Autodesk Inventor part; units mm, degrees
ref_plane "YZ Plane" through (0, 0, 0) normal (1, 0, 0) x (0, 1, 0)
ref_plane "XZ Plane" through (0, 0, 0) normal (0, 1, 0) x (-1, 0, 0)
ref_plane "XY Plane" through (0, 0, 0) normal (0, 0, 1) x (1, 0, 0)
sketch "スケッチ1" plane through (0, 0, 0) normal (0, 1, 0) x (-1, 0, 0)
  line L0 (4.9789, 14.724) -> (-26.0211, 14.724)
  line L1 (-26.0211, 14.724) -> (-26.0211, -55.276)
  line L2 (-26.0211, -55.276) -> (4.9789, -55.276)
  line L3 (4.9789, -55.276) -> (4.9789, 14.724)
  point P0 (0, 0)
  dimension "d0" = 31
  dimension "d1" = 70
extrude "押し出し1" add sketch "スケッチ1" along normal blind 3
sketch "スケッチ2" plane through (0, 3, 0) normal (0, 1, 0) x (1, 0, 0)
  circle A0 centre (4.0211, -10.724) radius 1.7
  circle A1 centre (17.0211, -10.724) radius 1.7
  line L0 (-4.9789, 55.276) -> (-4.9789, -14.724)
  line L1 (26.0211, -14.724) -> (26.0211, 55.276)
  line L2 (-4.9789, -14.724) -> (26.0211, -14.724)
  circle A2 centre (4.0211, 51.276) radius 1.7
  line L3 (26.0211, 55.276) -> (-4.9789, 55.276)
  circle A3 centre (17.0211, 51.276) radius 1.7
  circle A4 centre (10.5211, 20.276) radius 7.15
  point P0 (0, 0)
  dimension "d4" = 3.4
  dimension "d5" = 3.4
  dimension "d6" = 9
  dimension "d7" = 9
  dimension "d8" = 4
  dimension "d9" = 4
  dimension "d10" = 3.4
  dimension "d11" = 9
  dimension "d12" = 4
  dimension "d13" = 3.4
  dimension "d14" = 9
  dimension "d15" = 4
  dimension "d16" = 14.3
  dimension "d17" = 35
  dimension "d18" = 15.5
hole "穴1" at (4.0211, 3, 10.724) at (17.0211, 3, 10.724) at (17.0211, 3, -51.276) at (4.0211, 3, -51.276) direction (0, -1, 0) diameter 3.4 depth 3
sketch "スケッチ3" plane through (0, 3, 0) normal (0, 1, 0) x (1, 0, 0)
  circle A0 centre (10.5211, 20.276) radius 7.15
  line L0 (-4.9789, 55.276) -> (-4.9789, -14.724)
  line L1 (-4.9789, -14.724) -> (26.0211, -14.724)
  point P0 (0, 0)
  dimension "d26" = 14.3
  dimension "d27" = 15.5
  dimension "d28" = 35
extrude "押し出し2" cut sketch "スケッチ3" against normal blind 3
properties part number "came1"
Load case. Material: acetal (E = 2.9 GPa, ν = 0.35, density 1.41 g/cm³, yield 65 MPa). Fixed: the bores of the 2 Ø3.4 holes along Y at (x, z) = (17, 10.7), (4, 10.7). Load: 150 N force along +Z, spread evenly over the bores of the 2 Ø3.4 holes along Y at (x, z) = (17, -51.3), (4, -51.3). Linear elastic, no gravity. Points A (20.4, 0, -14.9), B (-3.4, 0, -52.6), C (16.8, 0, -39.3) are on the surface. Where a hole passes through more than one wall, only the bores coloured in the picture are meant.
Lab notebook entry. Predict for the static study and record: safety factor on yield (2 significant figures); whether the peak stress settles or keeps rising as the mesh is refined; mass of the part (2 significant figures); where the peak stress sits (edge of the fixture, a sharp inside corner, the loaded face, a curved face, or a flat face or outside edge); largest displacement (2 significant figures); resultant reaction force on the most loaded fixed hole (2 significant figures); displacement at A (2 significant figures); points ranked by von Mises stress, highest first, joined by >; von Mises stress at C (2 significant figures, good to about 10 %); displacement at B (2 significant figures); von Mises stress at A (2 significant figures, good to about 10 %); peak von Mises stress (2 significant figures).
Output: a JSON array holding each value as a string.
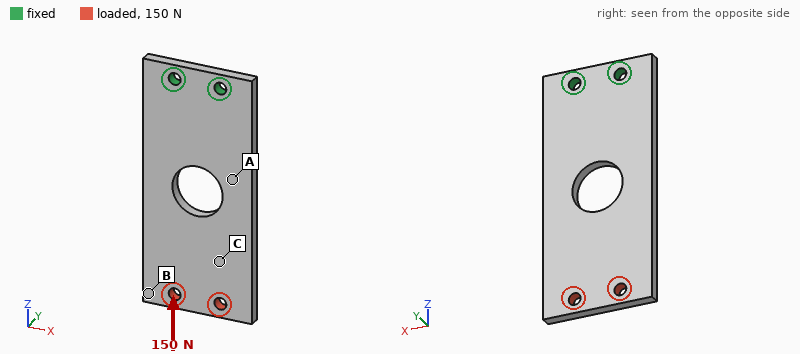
["9.7", "settles", "8.3 g", "a curved face", "56 µm", "75 N", "21 µm", "A > C > B", "1.8 MPa", "44 µm", "2.9 MPa", "6.7 MPa"]
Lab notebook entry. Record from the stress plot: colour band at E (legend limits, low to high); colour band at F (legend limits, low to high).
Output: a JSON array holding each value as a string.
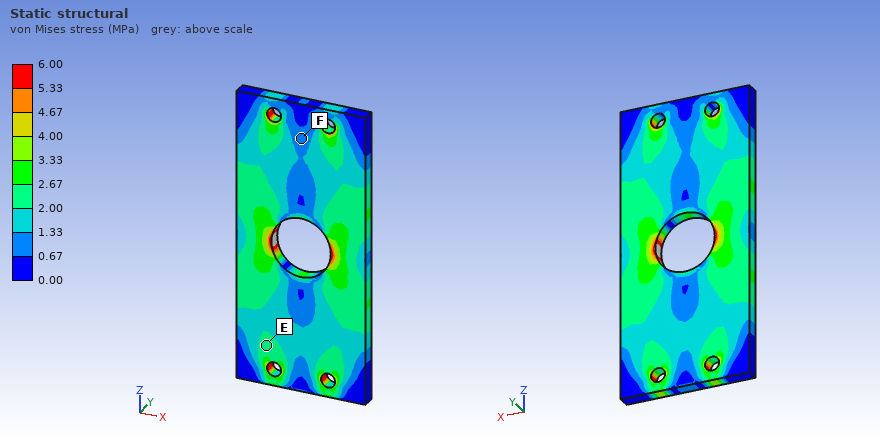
["2.00 to 2.67 MPa", "0.67 to 1.33 MPa"]
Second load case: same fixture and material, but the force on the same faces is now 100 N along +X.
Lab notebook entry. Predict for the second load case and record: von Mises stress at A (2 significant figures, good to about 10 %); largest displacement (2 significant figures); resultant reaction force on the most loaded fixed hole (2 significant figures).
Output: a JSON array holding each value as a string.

["6.4 MPa", "0.80 mm", "390 N"]
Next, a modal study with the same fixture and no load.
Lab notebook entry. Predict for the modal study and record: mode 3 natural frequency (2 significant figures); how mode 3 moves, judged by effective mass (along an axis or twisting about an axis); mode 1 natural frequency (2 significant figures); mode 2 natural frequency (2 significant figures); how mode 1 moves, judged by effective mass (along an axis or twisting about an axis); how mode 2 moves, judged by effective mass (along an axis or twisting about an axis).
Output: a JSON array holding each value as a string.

["980 Hz", "along Y", "160 Hz", "640 Hz", "along Y", "twisting about Z"]
